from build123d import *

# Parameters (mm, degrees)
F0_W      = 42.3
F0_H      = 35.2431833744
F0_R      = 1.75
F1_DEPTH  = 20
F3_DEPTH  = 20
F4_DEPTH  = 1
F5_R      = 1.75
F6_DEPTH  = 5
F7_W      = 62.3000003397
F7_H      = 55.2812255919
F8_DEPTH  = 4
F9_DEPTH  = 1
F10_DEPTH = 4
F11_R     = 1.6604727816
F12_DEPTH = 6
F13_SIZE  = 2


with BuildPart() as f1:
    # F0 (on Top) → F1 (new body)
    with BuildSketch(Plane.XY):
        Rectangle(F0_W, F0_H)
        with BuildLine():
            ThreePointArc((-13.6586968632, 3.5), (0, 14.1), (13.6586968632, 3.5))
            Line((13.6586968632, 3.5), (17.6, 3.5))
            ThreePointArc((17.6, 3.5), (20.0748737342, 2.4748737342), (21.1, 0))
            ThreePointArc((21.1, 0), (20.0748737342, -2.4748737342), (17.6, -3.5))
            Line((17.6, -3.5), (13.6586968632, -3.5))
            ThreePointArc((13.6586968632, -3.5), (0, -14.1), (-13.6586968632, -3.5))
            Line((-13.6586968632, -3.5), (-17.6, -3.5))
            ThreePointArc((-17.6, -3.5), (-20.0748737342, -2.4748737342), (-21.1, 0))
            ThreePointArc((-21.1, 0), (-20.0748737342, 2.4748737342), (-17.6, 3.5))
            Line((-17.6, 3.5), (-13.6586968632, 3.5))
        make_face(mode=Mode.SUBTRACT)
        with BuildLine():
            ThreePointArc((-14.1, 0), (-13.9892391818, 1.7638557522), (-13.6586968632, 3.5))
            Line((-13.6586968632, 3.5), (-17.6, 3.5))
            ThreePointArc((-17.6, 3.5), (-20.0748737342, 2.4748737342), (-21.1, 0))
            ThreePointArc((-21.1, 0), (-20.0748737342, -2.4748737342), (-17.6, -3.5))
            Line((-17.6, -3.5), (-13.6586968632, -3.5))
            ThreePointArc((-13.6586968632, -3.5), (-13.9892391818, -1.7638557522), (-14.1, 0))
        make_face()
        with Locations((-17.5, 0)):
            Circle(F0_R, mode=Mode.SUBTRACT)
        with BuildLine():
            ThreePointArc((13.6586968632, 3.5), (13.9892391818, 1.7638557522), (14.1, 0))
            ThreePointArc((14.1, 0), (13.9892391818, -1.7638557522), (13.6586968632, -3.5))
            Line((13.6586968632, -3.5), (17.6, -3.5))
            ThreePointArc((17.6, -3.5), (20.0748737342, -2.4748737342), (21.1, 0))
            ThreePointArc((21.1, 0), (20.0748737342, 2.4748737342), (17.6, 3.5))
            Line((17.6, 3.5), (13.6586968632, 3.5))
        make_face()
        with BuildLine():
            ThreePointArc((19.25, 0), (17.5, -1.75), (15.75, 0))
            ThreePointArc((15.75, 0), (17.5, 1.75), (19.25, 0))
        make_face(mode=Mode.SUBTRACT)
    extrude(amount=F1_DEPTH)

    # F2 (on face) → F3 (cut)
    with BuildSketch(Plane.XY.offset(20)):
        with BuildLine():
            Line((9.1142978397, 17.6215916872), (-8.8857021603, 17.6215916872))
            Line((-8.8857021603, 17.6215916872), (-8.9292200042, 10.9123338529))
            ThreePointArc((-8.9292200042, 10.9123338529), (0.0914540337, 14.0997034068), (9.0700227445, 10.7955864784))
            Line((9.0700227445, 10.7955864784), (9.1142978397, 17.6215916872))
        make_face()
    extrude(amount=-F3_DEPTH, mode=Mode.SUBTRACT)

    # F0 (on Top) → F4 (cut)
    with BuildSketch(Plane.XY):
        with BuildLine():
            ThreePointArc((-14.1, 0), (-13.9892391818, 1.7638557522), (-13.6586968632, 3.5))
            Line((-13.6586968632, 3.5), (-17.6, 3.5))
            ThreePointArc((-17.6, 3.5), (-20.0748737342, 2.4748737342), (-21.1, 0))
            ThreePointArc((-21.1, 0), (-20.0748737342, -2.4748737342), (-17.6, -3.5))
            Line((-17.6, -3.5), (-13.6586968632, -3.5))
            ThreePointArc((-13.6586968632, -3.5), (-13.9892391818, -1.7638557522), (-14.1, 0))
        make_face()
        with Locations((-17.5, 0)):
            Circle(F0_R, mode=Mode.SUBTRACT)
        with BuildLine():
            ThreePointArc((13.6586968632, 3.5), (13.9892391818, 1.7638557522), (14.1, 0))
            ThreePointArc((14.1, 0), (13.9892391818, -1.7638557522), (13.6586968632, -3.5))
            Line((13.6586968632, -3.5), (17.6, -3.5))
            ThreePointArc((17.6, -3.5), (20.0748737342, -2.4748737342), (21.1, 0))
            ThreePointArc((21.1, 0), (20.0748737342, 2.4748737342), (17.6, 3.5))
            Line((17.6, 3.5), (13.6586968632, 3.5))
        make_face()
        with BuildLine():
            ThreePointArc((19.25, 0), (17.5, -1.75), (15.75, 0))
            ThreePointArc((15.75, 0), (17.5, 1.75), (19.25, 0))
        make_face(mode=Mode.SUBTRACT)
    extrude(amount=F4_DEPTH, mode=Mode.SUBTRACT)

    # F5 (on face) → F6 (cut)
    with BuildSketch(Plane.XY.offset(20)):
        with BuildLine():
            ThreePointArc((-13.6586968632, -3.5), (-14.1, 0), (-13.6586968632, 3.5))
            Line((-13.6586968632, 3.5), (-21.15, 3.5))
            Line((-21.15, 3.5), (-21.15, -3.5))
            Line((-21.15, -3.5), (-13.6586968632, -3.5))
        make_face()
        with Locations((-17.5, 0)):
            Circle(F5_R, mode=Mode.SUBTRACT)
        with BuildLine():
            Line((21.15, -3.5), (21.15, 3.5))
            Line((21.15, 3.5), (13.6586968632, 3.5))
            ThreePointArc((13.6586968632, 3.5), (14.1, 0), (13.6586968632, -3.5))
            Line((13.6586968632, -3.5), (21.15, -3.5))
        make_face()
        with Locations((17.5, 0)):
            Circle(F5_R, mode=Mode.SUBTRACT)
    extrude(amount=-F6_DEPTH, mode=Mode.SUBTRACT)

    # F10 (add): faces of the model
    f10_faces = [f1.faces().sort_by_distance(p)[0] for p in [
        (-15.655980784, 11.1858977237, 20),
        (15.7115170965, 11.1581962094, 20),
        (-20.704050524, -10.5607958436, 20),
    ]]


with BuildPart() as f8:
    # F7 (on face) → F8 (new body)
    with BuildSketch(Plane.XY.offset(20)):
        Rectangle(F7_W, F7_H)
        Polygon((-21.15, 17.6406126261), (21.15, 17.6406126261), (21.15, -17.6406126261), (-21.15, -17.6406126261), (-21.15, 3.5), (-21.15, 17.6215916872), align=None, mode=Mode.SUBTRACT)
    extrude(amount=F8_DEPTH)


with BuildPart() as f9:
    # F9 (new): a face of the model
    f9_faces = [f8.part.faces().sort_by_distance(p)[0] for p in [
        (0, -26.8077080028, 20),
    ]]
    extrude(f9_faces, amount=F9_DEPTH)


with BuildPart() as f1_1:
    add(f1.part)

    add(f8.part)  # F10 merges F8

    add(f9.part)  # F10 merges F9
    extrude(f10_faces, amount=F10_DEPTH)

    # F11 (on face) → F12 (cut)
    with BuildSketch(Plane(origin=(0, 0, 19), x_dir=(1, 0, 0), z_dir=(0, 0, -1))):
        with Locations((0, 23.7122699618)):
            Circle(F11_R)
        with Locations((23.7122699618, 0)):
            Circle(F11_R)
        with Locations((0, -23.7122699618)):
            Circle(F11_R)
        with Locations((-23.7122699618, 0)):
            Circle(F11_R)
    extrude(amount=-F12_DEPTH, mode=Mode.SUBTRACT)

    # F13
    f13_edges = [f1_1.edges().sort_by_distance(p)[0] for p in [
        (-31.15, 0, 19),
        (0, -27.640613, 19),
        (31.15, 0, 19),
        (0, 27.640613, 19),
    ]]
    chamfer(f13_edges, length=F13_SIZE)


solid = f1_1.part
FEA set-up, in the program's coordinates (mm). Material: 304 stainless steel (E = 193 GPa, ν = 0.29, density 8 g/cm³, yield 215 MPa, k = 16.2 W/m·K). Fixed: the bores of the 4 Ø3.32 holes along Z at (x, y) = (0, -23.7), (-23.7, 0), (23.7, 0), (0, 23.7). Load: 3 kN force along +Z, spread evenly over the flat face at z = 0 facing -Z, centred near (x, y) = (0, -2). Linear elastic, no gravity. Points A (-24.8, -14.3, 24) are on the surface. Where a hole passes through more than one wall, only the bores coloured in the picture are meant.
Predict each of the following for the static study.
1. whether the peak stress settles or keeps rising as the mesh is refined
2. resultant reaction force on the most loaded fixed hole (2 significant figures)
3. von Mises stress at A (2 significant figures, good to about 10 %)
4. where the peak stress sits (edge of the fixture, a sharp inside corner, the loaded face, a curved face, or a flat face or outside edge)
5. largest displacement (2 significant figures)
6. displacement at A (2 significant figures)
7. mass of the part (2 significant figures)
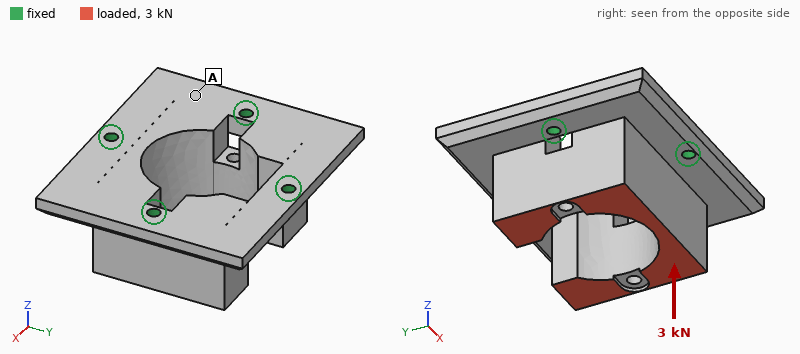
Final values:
keeps rising
1.4 kN
24 MPa
a sharp inside corner
14 µm
6.1 µm
210 g
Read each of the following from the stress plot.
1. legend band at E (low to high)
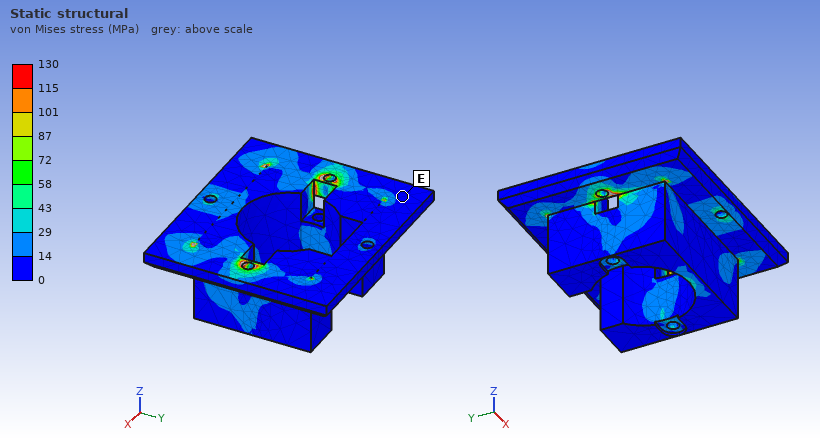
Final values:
0 to 14 MPa
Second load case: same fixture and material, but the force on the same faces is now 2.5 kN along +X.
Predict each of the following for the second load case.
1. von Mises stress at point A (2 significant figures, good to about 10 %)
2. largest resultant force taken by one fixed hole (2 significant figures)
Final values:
28 MPa
1.4 kN
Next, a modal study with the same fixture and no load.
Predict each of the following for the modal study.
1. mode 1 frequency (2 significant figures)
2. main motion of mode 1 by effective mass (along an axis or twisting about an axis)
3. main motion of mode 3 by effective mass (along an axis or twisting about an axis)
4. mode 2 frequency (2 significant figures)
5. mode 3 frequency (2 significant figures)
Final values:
4400 Hz
along Y
along Z
4900 Hz
6500 Hz
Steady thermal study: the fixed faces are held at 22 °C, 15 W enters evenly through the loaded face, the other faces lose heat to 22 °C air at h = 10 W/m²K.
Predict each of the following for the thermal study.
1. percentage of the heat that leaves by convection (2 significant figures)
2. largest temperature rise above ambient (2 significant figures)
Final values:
22 %
60 K
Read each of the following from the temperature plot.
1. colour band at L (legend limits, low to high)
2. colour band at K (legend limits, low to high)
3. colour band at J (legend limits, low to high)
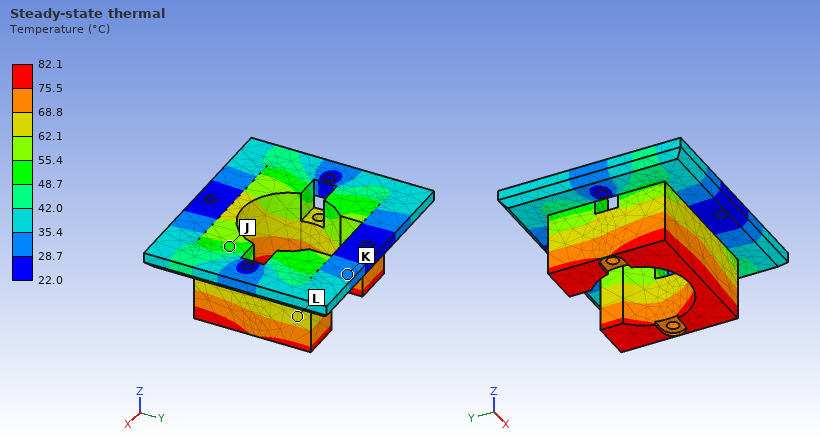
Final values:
62.1 to 68.8 °C
28.7 to 35.4 °C
48.7 to 55.4 °C
